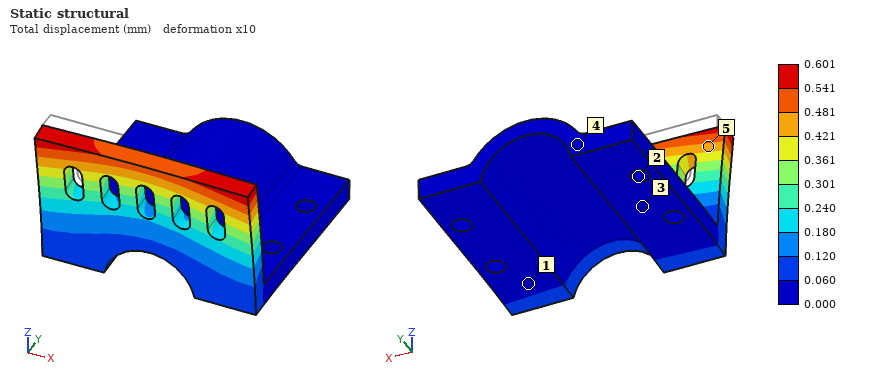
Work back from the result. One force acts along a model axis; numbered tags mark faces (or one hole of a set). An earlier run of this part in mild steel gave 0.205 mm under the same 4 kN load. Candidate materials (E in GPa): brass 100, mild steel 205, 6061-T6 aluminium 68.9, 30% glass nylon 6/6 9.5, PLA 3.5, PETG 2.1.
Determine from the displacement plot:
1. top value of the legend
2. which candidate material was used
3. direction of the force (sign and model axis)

0.601 mm
6061-T6 aluminium
-Y
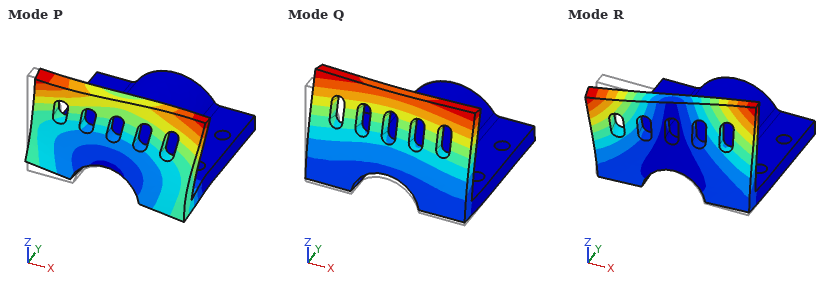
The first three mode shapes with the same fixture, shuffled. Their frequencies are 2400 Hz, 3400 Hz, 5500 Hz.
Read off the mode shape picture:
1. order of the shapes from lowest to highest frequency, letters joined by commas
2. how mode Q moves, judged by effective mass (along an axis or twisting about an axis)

Q, R, P
along Y
